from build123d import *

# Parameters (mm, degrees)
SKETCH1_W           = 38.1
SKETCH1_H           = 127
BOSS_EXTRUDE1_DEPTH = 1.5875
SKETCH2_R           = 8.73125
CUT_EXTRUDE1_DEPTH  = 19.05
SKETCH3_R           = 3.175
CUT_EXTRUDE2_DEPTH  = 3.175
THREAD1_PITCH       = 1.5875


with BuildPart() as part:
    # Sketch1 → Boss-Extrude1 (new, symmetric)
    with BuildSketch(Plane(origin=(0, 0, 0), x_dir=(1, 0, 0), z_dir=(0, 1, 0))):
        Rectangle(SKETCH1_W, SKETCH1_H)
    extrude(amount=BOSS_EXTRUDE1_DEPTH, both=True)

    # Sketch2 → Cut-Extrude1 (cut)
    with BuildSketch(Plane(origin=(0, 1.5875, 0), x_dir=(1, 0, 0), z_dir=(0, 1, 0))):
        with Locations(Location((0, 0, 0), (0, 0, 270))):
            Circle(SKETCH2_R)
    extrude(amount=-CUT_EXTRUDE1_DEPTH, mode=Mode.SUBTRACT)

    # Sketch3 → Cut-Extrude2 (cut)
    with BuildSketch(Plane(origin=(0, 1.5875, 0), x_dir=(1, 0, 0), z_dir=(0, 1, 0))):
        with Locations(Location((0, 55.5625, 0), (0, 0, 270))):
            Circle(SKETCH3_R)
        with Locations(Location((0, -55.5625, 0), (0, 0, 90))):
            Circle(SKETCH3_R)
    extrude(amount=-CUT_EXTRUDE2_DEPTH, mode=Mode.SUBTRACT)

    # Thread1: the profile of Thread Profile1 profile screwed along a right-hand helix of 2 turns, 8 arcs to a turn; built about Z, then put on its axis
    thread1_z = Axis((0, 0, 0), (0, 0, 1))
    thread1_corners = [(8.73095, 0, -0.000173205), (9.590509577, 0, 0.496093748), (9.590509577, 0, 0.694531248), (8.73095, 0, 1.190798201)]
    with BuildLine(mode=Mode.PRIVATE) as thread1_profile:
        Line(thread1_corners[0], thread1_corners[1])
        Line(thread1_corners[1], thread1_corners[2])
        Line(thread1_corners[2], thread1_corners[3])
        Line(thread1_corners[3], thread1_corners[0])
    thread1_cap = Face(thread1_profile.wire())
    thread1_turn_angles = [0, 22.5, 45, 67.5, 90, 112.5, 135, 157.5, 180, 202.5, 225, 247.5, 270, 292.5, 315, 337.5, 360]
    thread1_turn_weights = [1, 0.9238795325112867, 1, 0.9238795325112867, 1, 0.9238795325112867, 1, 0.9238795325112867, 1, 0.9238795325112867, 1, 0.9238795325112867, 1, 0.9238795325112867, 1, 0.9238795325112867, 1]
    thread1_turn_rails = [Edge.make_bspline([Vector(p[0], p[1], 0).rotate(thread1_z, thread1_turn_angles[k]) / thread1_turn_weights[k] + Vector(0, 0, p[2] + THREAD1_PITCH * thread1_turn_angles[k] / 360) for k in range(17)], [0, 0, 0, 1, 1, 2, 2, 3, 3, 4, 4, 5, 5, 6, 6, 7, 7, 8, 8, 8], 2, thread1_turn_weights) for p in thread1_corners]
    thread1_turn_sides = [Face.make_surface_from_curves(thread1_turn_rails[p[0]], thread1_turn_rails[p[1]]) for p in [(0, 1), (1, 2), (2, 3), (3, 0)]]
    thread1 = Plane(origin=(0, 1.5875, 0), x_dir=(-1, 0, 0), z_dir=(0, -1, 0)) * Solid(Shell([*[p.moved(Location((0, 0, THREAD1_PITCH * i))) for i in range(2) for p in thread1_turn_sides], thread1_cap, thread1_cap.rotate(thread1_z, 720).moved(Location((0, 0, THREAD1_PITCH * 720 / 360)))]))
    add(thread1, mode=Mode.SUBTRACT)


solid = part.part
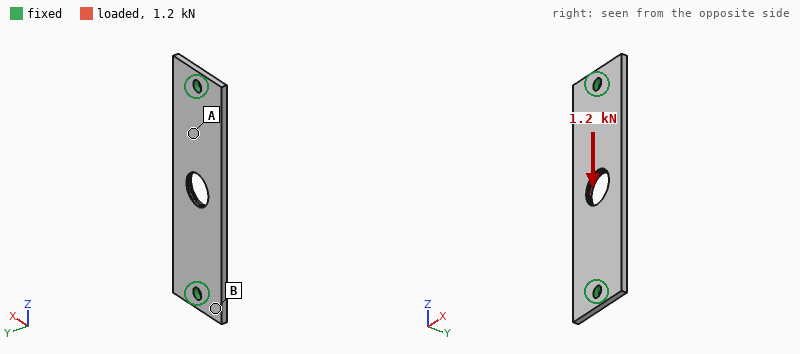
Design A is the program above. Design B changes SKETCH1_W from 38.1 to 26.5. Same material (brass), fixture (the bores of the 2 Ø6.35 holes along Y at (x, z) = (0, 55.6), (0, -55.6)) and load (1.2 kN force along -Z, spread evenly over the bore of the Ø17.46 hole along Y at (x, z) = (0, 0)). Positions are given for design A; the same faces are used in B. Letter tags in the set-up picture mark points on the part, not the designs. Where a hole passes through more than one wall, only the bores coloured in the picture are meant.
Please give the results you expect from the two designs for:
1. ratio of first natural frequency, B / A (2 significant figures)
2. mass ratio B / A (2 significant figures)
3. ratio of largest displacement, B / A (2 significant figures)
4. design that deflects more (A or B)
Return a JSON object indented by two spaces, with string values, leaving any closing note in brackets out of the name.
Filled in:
{
  "ratio of first natural frequency, B / A": "1.0",
  "mass ratio B / A": "0.67",
  "ratio of largest displacement, B / A": "1.5",
  "design that deflects more": "B"
}
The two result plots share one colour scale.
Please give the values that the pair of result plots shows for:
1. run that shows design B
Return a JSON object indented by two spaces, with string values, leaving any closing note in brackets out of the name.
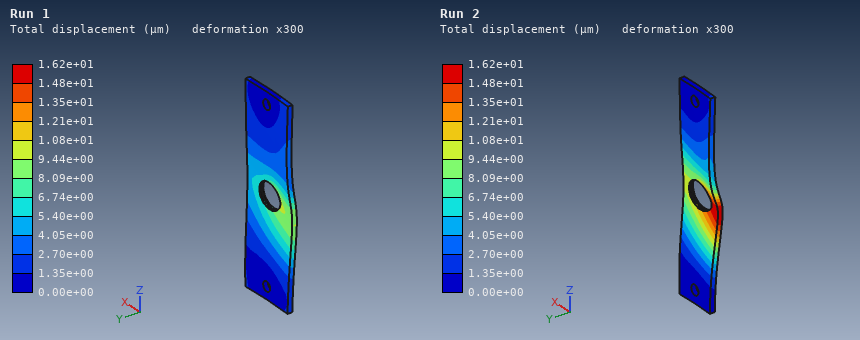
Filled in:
{
  "run that shows design B": "Run 2"
}
